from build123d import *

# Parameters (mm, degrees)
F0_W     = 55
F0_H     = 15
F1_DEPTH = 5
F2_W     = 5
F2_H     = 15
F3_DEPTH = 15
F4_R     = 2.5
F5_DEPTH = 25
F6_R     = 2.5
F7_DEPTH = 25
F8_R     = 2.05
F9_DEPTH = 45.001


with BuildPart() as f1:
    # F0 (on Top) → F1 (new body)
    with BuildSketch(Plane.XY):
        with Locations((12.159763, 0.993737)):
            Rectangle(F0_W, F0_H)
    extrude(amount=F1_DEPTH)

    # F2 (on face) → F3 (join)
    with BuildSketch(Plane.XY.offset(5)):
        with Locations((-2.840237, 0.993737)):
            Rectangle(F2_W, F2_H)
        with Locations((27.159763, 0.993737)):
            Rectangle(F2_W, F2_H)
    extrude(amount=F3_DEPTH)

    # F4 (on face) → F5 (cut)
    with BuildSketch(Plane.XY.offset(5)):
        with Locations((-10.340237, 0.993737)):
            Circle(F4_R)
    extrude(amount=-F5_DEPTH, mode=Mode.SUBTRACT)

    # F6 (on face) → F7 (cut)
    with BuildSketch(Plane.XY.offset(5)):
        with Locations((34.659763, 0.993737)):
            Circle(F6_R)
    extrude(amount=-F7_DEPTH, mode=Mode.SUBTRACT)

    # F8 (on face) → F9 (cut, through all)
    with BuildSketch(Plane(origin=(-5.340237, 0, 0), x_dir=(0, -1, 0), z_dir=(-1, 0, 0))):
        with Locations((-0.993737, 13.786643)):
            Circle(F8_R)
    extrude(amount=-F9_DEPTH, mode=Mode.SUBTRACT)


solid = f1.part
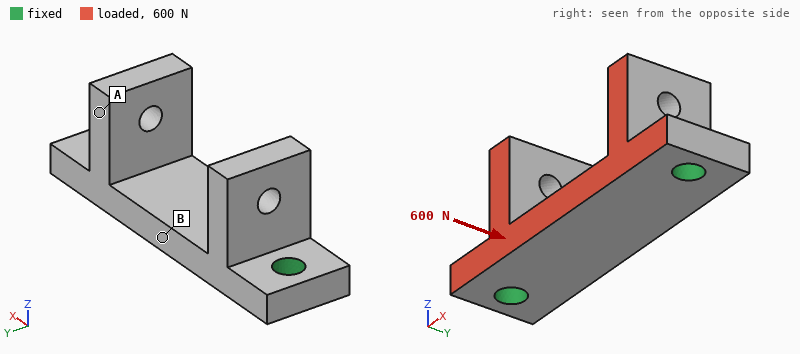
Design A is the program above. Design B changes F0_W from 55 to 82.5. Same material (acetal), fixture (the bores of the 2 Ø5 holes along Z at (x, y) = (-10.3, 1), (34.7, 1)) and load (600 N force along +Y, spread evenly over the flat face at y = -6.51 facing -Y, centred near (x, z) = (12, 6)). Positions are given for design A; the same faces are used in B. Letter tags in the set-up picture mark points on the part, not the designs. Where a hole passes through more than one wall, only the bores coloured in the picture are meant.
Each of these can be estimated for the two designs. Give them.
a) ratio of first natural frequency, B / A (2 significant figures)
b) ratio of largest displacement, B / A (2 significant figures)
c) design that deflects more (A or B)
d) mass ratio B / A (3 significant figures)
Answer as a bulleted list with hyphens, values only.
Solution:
- 1.0
- 0.70
- A
- 1.34
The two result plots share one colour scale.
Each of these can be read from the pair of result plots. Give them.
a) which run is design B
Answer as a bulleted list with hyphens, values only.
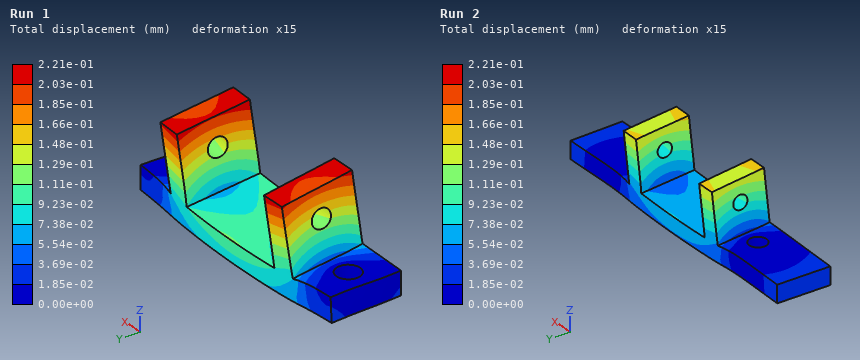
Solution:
- Run 2
